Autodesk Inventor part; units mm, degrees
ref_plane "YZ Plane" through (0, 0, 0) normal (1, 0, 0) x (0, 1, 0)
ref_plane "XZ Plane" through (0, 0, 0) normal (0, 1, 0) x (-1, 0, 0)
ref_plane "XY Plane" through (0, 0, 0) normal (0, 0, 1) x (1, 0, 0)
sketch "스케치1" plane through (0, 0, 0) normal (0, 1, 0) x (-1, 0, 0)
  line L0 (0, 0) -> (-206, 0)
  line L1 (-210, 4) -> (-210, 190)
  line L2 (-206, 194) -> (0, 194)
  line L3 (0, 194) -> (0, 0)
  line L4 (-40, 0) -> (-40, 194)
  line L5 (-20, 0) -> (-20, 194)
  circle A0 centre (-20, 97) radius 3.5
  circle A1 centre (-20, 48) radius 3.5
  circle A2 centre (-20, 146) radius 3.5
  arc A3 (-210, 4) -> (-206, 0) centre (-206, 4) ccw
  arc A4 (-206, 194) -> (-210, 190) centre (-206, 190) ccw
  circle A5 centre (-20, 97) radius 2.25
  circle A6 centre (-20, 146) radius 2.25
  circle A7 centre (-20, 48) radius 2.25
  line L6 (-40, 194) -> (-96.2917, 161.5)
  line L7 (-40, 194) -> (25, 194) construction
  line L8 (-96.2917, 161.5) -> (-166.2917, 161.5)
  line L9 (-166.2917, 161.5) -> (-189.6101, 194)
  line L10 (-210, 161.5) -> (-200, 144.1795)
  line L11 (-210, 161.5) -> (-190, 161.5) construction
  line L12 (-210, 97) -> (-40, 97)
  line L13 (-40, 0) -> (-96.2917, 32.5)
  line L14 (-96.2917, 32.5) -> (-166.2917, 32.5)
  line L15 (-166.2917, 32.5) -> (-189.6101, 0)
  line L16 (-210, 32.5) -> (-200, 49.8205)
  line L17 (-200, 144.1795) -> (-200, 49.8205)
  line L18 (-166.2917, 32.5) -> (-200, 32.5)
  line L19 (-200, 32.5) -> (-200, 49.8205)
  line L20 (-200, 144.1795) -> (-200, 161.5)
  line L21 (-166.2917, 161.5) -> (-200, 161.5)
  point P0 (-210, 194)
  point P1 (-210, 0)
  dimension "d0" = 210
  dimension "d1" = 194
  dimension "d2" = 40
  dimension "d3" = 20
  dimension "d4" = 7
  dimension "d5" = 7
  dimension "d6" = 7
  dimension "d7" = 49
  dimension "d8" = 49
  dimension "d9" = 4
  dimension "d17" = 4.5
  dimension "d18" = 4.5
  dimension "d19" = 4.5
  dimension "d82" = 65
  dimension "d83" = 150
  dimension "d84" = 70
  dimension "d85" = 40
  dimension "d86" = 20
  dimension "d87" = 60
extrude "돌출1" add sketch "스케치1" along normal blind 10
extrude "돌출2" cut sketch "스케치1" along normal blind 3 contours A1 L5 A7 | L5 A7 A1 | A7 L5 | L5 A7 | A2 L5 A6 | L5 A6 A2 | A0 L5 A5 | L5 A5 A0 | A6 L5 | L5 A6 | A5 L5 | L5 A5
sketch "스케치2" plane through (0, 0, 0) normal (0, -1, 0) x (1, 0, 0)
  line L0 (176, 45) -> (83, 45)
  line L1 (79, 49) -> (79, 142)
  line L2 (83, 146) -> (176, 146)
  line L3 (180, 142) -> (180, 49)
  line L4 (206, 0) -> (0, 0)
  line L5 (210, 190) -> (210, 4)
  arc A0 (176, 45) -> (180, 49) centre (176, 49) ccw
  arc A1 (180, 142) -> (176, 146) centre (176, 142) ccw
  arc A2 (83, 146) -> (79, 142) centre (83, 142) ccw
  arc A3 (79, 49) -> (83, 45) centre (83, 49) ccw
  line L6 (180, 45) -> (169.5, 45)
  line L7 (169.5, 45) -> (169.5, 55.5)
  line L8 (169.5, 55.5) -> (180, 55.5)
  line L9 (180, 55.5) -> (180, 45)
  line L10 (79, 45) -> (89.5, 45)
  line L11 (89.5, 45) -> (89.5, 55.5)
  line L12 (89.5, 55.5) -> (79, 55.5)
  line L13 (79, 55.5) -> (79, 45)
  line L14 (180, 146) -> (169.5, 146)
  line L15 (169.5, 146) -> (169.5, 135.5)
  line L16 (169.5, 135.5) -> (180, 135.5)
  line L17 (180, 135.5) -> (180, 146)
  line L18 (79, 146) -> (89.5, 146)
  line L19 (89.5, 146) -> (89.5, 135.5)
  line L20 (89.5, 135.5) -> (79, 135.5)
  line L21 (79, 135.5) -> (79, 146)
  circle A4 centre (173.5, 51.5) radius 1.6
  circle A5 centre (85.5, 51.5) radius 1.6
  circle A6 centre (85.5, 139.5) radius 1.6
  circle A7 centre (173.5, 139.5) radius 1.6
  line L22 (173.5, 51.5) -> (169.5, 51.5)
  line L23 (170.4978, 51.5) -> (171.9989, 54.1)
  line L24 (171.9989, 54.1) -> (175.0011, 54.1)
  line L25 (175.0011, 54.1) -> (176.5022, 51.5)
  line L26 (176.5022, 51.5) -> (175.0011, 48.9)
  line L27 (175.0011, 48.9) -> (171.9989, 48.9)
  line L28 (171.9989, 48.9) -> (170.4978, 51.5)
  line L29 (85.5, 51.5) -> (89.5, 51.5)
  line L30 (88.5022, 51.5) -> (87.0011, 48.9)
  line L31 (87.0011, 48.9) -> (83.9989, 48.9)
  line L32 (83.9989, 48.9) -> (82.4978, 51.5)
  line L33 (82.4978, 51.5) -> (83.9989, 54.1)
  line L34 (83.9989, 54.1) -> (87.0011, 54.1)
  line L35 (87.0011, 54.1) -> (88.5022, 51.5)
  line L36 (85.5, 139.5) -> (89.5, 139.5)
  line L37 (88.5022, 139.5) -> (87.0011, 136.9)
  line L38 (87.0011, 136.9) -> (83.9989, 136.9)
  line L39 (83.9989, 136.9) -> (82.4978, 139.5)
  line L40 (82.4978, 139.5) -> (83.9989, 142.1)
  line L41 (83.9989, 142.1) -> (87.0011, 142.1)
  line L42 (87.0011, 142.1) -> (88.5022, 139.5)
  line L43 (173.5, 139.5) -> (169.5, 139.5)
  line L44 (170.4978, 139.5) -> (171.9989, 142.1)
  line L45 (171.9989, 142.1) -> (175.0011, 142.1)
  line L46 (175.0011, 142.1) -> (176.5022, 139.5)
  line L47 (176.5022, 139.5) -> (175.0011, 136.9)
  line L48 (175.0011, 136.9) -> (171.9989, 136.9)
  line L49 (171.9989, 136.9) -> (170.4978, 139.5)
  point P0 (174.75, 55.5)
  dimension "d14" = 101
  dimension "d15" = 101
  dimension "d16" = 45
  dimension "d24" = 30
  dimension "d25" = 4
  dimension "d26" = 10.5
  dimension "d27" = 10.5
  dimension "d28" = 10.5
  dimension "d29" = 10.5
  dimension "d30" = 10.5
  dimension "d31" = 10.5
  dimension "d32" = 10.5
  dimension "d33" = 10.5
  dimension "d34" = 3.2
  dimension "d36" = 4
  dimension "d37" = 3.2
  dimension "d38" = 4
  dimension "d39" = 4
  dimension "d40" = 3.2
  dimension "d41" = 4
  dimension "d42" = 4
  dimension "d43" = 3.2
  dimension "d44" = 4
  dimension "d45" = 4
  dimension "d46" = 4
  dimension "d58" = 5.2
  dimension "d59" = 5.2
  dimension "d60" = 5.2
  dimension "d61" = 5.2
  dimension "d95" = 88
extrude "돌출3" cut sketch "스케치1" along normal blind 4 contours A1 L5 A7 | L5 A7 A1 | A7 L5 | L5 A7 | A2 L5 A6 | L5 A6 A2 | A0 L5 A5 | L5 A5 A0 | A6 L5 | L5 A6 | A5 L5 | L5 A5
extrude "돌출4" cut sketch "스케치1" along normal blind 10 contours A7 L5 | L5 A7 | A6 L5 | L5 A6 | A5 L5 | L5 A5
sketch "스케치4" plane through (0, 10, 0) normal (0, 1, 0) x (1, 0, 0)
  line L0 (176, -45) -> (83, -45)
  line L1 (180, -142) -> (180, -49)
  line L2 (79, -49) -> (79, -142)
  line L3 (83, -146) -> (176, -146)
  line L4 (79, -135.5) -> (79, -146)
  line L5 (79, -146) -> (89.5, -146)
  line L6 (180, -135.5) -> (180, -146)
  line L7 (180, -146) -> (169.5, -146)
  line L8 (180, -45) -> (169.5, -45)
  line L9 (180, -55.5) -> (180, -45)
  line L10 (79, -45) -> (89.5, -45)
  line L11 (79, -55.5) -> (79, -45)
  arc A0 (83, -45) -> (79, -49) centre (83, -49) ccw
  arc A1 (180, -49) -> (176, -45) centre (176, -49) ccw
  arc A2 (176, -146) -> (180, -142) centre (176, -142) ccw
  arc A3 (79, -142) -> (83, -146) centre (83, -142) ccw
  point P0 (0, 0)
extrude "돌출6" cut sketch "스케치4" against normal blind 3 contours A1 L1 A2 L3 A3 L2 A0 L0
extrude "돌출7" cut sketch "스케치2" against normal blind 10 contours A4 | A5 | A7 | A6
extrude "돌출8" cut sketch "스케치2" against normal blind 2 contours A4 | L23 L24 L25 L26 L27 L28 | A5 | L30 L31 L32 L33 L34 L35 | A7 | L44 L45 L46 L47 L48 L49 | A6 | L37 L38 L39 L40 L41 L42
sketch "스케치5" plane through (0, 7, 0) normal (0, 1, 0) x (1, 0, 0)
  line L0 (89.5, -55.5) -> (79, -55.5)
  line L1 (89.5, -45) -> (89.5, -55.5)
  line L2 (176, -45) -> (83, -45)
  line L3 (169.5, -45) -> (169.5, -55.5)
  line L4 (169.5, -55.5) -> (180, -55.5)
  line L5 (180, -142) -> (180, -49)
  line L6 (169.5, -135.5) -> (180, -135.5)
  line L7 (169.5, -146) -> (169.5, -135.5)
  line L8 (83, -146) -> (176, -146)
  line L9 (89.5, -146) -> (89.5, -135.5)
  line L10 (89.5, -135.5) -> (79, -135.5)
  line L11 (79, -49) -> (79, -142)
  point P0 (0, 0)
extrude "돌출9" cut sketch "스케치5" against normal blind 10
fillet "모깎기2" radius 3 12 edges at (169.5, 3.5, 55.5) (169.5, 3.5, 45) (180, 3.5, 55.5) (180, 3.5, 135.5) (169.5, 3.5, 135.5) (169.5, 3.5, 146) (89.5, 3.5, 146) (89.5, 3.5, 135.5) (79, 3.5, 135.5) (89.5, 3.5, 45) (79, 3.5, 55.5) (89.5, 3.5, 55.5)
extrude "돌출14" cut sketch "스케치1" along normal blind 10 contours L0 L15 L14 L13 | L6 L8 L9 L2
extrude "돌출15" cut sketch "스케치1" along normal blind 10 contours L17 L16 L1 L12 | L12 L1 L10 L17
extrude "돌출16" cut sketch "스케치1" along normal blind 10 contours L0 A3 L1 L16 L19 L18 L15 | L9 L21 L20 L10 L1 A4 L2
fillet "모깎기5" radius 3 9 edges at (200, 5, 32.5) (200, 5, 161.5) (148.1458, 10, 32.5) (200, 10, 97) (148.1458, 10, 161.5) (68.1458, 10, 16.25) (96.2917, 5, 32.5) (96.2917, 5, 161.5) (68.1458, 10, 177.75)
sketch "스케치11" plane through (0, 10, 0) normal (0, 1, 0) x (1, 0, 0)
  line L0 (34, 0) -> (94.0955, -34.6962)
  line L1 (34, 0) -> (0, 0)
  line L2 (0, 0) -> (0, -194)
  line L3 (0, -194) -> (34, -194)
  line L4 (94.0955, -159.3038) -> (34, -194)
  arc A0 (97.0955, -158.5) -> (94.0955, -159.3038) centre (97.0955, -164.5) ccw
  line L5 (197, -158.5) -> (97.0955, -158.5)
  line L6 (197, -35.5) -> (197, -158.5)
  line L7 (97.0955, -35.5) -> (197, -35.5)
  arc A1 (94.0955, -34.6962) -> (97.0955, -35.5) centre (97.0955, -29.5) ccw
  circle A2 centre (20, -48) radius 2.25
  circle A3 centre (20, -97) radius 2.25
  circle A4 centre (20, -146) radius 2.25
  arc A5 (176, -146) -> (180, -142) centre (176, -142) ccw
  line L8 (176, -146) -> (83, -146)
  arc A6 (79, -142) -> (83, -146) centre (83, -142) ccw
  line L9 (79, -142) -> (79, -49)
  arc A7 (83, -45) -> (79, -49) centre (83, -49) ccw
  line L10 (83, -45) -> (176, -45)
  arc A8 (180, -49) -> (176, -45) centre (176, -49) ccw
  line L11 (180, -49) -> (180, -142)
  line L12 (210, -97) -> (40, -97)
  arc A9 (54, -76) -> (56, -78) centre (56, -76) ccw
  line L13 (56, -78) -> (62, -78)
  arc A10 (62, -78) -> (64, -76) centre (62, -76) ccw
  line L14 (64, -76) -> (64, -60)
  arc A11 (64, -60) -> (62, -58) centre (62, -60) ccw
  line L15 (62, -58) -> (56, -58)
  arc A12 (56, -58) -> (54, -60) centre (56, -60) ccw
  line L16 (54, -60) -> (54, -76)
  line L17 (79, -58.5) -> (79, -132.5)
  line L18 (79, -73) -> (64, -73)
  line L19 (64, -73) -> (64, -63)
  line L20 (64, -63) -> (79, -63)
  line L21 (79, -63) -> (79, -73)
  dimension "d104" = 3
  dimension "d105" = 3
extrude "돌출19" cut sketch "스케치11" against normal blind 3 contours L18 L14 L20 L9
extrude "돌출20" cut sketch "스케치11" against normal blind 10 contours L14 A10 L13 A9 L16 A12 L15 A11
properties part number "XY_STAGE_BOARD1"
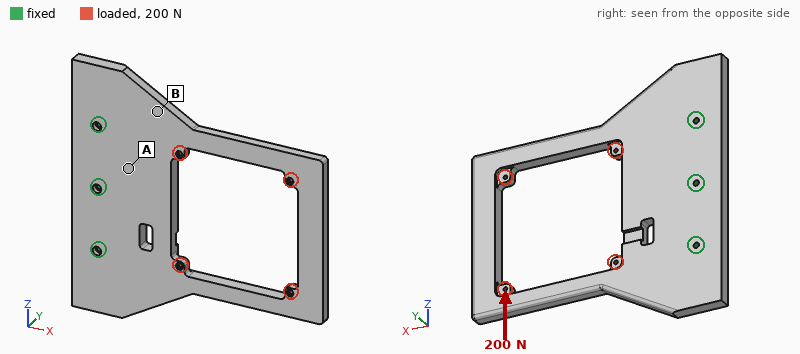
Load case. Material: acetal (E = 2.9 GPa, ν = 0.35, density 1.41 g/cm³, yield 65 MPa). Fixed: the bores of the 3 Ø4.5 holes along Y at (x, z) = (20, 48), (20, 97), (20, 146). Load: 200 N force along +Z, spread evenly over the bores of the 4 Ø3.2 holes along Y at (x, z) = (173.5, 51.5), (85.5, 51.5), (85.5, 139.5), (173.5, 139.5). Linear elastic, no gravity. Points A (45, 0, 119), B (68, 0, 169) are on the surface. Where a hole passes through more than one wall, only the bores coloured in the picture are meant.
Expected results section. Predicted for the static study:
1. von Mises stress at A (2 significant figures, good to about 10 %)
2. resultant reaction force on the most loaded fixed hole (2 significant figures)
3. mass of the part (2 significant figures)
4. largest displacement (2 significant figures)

0.58 MPa
240 N
280 g
0.70 mm
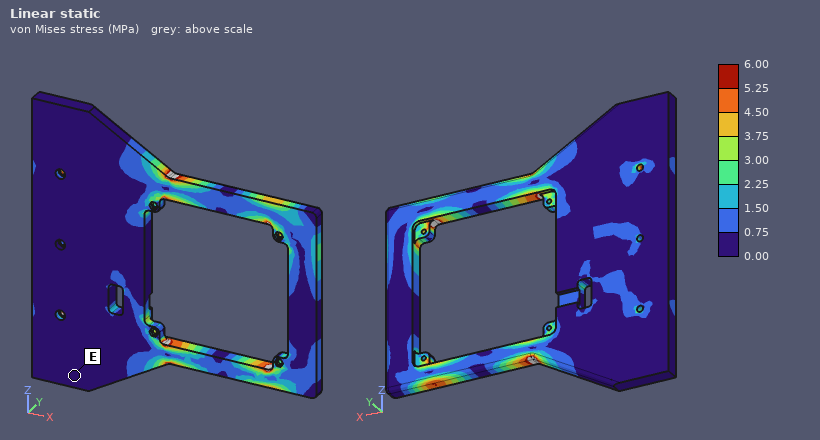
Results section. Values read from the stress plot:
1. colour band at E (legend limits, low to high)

0.00 to 0.75 MPa
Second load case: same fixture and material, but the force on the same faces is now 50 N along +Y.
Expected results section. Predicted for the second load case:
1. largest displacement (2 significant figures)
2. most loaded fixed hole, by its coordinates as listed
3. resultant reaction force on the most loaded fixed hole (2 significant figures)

3.3 mm
(20, 97)
28 N
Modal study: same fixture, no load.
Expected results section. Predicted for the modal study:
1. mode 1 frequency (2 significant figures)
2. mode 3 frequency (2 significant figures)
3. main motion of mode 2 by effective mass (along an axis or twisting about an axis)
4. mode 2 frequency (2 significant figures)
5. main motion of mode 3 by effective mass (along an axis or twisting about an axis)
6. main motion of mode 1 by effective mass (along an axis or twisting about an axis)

66 Hz
270 Hz
twisting about X
170 Hz
along Z
along Y
